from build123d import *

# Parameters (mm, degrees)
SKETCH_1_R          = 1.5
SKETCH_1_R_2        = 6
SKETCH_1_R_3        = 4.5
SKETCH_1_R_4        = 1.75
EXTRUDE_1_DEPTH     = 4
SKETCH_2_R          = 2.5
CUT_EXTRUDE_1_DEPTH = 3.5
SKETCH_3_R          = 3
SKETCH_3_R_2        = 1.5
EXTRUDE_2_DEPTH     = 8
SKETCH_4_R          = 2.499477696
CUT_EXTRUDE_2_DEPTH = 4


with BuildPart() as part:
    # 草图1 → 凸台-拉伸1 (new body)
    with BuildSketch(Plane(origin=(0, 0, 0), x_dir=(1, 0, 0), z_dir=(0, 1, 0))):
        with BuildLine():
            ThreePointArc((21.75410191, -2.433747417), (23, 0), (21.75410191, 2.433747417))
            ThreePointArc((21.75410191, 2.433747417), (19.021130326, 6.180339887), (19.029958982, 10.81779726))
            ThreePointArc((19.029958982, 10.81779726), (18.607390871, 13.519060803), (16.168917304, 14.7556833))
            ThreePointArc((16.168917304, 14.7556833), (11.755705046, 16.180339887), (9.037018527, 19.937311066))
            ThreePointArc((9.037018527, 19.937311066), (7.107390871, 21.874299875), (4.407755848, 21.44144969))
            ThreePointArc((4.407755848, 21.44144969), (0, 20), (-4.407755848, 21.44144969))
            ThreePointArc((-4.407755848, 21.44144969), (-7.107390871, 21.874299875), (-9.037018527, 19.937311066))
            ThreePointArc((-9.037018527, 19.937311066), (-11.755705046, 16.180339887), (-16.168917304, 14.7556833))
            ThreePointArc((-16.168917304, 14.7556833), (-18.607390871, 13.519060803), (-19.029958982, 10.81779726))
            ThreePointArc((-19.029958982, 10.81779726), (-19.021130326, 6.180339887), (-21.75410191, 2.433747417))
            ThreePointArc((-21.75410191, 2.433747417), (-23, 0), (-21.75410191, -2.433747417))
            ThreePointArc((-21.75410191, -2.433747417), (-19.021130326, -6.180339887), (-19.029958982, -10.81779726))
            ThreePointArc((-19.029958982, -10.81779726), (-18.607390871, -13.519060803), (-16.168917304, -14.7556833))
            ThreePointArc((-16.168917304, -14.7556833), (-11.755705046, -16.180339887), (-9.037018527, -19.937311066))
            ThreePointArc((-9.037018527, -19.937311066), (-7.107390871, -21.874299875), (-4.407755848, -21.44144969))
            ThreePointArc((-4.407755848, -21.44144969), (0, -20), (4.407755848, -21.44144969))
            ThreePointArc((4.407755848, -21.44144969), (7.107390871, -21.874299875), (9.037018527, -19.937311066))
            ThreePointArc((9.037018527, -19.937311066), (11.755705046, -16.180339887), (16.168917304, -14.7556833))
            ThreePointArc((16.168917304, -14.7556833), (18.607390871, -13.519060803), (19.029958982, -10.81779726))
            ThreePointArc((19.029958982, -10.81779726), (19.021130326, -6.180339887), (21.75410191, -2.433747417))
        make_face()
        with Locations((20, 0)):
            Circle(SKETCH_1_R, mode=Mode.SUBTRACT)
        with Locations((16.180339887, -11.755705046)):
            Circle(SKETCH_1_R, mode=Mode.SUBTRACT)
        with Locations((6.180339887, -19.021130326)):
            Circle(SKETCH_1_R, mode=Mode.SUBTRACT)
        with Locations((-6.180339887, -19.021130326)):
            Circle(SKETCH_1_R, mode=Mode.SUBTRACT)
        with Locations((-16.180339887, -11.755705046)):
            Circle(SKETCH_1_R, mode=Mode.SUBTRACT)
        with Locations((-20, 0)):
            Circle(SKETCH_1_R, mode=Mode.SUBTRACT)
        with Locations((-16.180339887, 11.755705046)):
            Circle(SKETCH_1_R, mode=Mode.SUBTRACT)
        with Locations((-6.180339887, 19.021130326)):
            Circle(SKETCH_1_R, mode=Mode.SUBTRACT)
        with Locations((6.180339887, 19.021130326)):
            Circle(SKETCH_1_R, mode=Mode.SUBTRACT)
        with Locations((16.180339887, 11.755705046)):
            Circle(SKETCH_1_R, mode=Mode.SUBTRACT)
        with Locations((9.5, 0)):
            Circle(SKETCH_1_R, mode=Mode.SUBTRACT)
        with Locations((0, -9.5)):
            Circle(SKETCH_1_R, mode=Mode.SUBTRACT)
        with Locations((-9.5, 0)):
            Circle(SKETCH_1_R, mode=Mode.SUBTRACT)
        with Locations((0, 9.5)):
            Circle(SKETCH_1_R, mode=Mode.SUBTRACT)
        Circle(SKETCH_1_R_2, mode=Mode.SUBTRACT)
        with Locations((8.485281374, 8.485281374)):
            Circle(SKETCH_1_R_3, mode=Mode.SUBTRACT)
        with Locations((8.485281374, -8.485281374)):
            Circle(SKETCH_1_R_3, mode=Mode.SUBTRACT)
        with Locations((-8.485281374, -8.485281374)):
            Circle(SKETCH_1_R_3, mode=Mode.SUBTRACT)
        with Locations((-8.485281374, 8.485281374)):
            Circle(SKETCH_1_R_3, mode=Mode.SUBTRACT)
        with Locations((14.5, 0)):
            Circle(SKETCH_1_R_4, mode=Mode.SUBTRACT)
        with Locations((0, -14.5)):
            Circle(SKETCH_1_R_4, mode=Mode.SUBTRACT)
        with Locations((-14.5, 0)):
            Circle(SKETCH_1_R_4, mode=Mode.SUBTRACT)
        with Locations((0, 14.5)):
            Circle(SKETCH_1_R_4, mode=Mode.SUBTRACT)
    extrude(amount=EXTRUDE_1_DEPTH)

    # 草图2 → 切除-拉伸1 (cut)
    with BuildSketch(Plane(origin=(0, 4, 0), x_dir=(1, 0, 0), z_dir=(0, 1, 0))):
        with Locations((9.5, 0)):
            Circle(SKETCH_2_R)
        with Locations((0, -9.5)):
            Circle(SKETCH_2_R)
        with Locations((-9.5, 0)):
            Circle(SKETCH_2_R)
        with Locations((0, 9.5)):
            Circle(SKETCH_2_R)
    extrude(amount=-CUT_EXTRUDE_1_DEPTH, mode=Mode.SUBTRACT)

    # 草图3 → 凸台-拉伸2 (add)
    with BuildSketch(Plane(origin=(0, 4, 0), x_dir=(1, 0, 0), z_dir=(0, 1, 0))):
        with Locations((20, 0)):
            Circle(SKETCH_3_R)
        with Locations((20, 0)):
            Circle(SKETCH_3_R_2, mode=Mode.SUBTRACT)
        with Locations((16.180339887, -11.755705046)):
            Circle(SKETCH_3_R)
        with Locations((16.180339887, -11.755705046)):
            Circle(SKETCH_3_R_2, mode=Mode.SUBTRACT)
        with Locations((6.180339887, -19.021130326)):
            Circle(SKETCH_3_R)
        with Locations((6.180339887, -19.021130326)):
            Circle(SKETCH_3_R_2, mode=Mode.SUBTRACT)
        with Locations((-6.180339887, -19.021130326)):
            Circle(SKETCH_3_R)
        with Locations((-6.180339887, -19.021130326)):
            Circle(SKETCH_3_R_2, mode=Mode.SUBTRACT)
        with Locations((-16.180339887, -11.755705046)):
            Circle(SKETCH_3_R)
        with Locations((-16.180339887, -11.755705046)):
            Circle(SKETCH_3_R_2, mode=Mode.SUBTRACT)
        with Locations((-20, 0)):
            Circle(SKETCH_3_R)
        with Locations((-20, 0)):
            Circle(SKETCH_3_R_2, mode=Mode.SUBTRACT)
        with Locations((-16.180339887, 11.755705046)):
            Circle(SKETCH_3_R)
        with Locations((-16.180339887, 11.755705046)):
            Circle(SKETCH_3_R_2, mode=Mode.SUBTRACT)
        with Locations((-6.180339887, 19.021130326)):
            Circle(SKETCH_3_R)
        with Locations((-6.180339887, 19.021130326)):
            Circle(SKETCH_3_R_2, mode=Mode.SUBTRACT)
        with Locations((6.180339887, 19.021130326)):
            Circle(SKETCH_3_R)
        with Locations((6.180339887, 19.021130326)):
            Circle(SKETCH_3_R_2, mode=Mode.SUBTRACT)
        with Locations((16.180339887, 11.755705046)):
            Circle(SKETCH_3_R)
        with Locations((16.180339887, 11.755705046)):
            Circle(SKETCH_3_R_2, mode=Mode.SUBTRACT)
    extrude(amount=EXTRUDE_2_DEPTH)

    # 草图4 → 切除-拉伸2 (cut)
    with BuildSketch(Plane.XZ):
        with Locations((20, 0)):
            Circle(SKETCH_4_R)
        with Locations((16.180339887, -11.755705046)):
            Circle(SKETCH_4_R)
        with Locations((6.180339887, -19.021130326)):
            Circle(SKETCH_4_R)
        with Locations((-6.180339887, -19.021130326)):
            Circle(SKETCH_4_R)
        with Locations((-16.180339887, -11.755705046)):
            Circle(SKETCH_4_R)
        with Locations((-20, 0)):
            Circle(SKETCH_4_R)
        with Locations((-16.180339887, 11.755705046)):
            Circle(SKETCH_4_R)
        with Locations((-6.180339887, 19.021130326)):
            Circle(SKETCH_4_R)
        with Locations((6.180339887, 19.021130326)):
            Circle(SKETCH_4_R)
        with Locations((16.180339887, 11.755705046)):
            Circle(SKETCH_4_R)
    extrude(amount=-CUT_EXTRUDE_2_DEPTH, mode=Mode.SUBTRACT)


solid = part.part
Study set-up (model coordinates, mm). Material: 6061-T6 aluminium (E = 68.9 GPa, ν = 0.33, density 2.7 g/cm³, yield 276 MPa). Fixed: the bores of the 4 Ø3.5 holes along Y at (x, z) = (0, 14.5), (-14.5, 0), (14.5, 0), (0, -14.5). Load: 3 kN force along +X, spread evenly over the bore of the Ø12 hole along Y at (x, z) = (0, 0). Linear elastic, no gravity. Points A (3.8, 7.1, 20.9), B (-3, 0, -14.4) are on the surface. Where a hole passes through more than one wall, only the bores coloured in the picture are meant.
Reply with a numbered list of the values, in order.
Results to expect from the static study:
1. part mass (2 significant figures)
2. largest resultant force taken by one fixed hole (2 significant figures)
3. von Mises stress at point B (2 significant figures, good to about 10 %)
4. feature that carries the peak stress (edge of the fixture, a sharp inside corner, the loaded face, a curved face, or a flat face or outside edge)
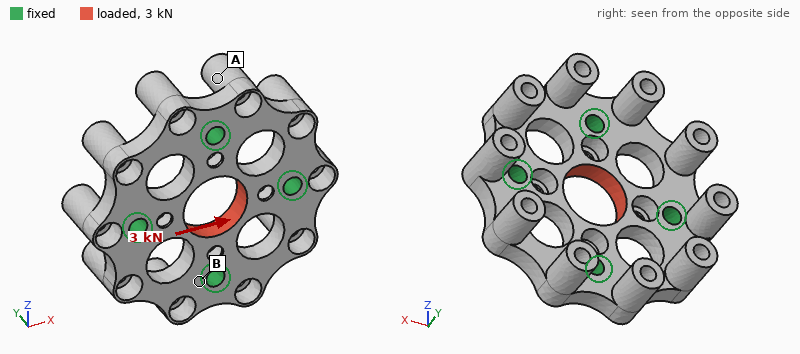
1. 13 g
2. 1.1 kN
3. 21 MPa
4. a curved face
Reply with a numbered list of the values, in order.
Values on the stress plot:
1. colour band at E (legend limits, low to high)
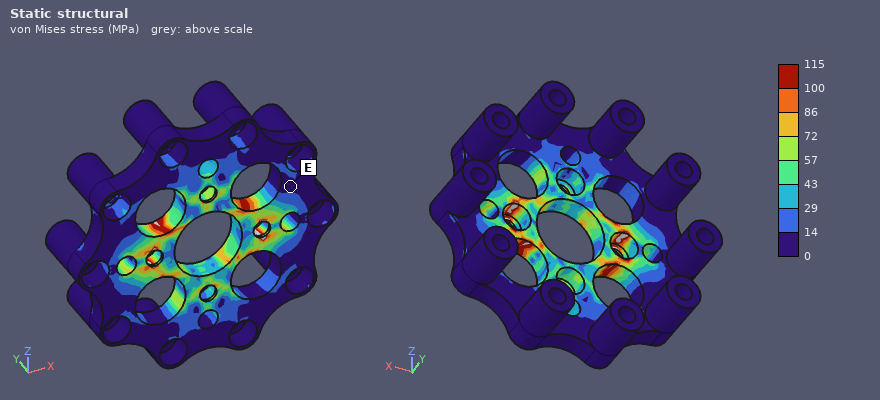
1. 0 to 14 MPa
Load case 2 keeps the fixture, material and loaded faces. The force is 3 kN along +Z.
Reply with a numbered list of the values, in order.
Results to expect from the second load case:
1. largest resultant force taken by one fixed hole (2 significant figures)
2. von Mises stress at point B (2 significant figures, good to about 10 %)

1. 1.1 kN
2. 35 MPa
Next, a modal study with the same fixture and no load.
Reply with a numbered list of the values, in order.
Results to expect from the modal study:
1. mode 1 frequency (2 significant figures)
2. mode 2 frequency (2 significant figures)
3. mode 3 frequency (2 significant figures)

1. 13 kHz
2. 13 kHz
3. 13 kHz
